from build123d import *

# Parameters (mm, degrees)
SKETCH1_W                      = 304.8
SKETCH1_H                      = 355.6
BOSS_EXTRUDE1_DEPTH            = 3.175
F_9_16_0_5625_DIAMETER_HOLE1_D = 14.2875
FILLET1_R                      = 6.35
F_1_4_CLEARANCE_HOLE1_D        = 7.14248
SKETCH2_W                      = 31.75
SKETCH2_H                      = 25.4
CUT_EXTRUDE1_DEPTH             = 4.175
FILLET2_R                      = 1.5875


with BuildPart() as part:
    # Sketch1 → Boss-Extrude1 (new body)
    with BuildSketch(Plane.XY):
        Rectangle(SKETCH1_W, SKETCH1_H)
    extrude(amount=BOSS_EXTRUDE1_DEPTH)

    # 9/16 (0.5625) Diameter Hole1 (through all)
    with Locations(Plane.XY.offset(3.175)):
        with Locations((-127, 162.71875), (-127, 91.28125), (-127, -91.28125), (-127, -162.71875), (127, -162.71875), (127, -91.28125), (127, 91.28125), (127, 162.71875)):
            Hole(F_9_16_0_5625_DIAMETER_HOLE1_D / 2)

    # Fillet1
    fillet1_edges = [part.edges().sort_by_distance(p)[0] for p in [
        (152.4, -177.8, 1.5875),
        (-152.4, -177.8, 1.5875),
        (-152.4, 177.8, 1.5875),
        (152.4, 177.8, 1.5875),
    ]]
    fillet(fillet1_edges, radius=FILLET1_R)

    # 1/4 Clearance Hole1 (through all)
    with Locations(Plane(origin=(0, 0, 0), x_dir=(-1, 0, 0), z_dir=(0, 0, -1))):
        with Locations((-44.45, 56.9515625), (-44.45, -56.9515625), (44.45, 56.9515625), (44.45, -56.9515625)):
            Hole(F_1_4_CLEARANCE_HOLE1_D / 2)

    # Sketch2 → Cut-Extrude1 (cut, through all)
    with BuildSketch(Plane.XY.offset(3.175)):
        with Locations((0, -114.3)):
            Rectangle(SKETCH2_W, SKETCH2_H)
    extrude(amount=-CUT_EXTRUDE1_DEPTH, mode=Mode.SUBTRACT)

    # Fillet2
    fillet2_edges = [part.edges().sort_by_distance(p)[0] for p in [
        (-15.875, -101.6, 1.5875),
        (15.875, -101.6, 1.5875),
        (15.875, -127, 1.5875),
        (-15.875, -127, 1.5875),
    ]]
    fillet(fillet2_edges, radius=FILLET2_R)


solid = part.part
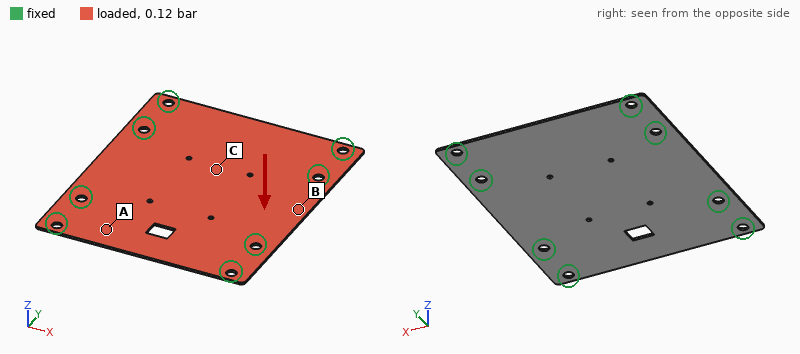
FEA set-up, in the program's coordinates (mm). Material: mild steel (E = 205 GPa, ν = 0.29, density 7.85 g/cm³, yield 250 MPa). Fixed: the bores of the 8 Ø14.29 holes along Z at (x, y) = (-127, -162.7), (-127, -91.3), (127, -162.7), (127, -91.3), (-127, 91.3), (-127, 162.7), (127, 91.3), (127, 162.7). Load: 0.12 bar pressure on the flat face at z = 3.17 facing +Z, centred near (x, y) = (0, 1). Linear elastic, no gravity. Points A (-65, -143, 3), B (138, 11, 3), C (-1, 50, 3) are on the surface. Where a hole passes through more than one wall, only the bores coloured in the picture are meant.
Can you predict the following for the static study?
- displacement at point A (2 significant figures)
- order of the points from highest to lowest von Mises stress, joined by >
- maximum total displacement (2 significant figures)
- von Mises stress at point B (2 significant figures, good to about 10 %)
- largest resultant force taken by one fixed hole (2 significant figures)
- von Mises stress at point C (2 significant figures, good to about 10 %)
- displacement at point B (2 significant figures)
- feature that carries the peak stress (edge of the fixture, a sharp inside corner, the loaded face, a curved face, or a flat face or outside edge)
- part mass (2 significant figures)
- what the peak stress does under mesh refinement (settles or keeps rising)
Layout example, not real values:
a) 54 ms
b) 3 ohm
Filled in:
a) 0.12 mm
b) C > B > A
c) 0.32 mm
d) 11 MPa
e) 240 N
f) 18 MPa
g) 0.056 mm
h) edge of the fixture
i) 2.6 kg
j) keeps rising
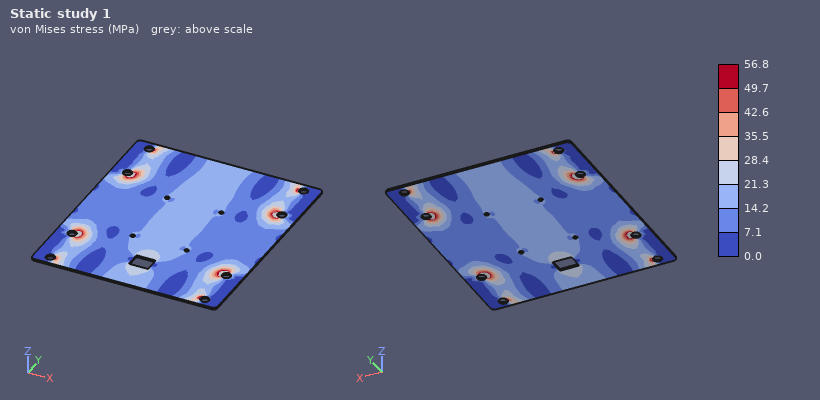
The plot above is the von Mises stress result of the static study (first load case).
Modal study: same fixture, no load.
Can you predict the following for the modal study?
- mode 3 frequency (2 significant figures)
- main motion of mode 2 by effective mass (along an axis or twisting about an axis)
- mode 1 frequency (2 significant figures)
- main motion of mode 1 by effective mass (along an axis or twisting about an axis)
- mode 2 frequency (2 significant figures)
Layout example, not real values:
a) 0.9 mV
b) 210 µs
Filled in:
a) 370 Hz
b) twisting about X
c) 240 Hz
d) along Z
e) 300 Hz
